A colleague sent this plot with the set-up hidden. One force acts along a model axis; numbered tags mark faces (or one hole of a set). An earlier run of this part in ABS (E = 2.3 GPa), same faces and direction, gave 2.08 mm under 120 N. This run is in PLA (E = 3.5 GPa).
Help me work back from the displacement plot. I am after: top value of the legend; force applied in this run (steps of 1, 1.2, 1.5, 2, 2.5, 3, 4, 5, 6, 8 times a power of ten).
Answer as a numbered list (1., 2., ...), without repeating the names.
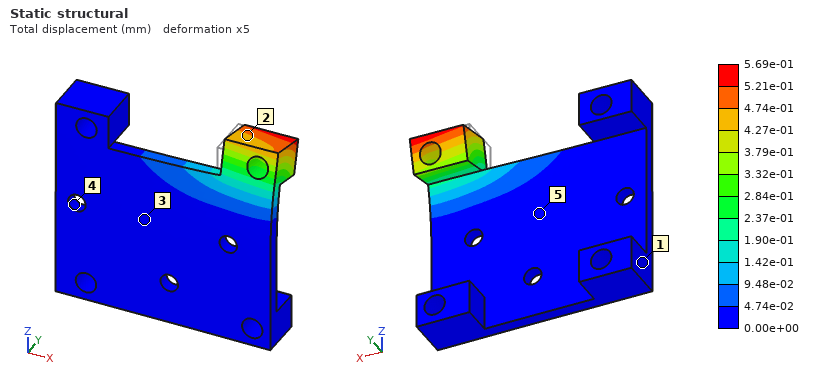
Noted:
1. 5.69e-01 mm
2. 50 N
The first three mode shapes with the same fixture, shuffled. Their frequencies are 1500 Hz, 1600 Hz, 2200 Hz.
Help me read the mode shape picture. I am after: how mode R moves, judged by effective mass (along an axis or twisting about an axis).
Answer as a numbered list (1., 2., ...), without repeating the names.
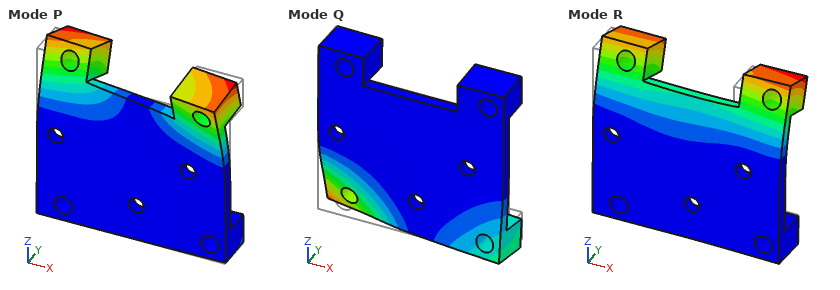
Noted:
1. along Y
